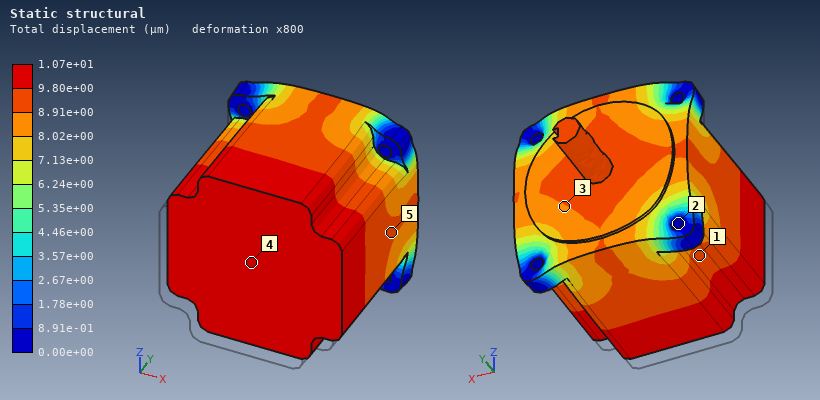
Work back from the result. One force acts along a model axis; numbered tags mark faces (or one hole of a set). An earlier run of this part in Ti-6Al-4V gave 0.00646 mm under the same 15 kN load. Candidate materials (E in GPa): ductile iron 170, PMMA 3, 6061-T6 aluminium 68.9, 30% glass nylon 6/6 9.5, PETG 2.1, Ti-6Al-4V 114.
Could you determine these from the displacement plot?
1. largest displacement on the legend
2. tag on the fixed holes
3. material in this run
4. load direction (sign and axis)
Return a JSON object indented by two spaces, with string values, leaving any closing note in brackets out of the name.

{
  "largest displacement on the legend": "1.07e+01 µm",
  "tag on the fixed holes": "2",
  "material in this run": "6061-T6 aluminium",
  "load direction": "+Y"
}
